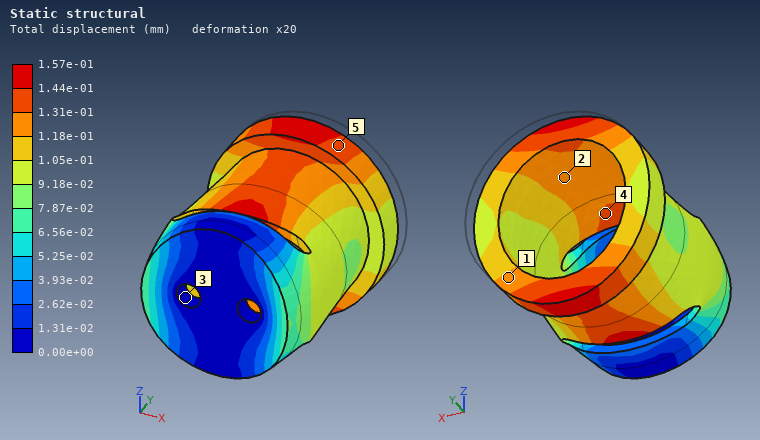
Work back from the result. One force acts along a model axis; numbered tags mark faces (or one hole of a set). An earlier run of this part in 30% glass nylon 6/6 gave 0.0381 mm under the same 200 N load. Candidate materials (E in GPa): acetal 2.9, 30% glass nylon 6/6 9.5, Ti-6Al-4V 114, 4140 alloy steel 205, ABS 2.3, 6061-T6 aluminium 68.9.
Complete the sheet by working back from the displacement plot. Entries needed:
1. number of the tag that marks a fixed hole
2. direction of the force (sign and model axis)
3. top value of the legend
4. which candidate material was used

3
-Y
1.57e-01 mm
ABS
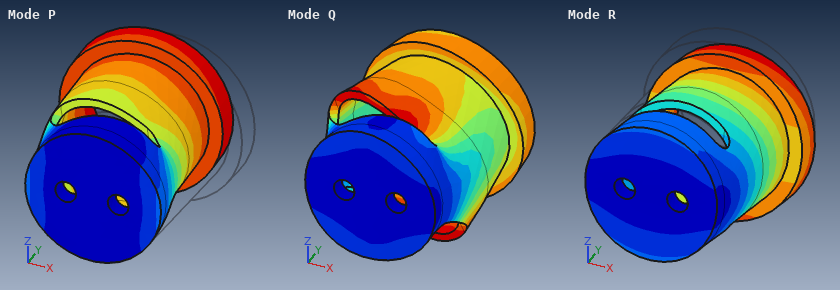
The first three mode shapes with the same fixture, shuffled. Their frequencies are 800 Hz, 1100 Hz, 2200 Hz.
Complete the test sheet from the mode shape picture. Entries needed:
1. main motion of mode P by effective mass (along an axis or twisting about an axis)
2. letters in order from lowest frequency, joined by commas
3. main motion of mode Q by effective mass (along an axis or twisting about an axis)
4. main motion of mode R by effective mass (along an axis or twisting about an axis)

along X
R, P, Q
twisting about Y
along Z
